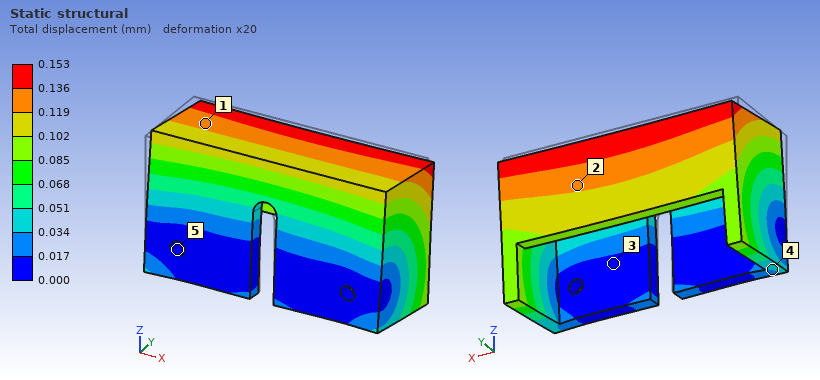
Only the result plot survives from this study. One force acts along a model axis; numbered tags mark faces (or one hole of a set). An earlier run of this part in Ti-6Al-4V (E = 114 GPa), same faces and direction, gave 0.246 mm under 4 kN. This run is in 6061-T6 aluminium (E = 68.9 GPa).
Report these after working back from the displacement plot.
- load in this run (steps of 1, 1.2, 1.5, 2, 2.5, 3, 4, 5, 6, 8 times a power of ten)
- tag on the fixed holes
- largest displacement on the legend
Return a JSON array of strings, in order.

["1.5 kN", "5", "0.153 mm"]
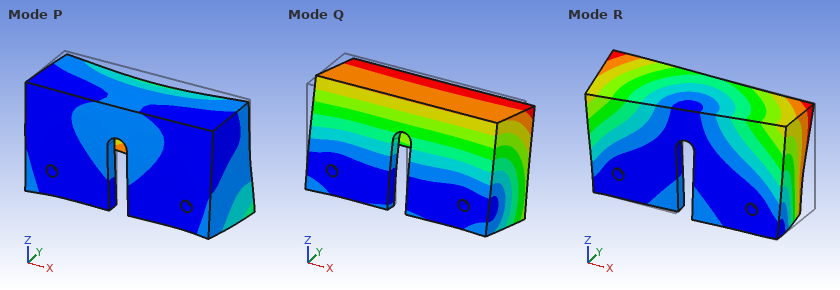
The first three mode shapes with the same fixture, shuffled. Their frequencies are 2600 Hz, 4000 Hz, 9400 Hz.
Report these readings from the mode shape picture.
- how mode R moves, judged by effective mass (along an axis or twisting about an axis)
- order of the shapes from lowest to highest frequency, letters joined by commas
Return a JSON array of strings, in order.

["along X", "Q, R, P"]
